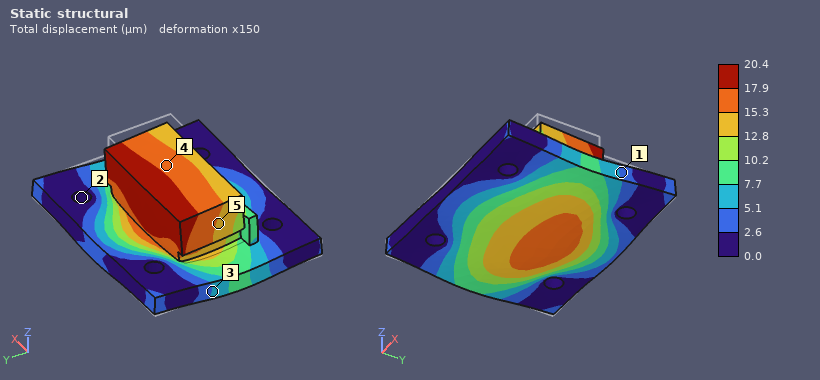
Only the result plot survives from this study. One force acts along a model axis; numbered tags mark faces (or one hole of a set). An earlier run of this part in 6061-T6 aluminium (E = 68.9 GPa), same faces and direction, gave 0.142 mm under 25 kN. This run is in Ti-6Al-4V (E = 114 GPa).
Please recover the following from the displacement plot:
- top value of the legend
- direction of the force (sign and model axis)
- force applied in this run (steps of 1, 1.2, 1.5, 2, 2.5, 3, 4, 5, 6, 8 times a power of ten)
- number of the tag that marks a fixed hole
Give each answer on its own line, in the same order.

20.4 µm
-Z
6 kN
2
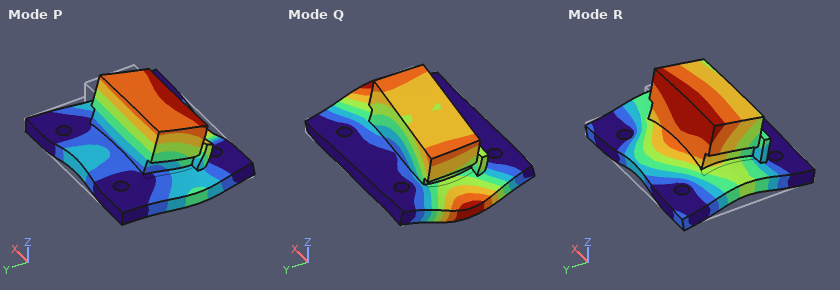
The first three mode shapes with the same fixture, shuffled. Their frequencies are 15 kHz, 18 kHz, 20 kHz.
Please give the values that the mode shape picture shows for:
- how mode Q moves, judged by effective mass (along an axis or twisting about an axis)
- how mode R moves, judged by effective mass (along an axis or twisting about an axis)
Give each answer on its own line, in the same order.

along X
along Z
